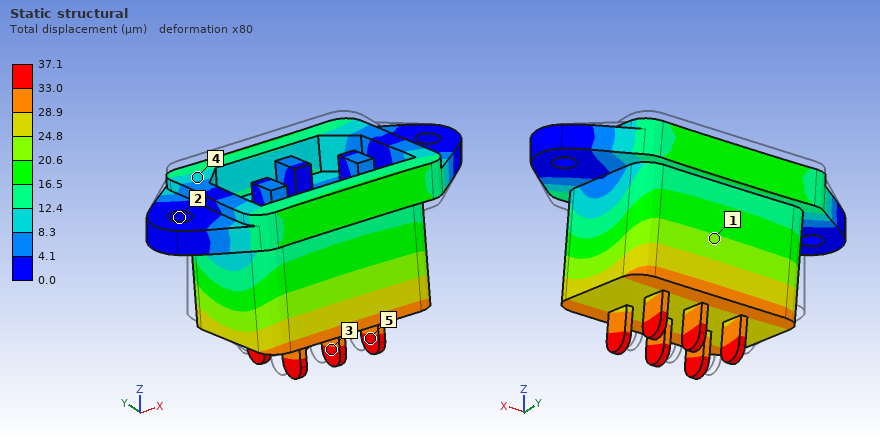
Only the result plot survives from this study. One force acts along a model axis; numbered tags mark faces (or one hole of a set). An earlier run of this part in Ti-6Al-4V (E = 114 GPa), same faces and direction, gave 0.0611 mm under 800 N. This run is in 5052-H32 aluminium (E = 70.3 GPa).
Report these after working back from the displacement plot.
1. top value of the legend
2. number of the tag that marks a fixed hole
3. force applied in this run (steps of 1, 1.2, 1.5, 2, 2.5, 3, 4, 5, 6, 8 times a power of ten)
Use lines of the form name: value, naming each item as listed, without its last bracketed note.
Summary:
top value of the legend: 37.1 µm
number of the tag that marks a fixed hole: 2
force applied in this run: 300 N
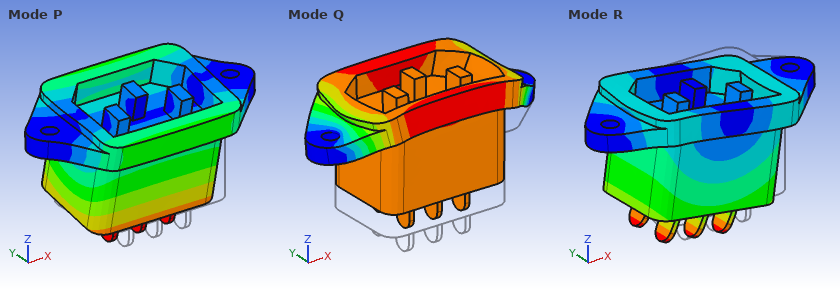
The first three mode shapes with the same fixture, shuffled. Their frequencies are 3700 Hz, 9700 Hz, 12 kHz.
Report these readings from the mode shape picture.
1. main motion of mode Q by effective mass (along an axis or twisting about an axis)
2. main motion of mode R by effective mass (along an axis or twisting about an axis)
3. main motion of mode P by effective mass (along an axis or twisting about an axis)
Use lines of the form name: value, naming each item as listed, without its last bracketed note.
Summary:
main motion of mode Q by effective mass: along Z
main motion of mode R by effective mass: along X
main motion of mode P by effective mass: along Y
